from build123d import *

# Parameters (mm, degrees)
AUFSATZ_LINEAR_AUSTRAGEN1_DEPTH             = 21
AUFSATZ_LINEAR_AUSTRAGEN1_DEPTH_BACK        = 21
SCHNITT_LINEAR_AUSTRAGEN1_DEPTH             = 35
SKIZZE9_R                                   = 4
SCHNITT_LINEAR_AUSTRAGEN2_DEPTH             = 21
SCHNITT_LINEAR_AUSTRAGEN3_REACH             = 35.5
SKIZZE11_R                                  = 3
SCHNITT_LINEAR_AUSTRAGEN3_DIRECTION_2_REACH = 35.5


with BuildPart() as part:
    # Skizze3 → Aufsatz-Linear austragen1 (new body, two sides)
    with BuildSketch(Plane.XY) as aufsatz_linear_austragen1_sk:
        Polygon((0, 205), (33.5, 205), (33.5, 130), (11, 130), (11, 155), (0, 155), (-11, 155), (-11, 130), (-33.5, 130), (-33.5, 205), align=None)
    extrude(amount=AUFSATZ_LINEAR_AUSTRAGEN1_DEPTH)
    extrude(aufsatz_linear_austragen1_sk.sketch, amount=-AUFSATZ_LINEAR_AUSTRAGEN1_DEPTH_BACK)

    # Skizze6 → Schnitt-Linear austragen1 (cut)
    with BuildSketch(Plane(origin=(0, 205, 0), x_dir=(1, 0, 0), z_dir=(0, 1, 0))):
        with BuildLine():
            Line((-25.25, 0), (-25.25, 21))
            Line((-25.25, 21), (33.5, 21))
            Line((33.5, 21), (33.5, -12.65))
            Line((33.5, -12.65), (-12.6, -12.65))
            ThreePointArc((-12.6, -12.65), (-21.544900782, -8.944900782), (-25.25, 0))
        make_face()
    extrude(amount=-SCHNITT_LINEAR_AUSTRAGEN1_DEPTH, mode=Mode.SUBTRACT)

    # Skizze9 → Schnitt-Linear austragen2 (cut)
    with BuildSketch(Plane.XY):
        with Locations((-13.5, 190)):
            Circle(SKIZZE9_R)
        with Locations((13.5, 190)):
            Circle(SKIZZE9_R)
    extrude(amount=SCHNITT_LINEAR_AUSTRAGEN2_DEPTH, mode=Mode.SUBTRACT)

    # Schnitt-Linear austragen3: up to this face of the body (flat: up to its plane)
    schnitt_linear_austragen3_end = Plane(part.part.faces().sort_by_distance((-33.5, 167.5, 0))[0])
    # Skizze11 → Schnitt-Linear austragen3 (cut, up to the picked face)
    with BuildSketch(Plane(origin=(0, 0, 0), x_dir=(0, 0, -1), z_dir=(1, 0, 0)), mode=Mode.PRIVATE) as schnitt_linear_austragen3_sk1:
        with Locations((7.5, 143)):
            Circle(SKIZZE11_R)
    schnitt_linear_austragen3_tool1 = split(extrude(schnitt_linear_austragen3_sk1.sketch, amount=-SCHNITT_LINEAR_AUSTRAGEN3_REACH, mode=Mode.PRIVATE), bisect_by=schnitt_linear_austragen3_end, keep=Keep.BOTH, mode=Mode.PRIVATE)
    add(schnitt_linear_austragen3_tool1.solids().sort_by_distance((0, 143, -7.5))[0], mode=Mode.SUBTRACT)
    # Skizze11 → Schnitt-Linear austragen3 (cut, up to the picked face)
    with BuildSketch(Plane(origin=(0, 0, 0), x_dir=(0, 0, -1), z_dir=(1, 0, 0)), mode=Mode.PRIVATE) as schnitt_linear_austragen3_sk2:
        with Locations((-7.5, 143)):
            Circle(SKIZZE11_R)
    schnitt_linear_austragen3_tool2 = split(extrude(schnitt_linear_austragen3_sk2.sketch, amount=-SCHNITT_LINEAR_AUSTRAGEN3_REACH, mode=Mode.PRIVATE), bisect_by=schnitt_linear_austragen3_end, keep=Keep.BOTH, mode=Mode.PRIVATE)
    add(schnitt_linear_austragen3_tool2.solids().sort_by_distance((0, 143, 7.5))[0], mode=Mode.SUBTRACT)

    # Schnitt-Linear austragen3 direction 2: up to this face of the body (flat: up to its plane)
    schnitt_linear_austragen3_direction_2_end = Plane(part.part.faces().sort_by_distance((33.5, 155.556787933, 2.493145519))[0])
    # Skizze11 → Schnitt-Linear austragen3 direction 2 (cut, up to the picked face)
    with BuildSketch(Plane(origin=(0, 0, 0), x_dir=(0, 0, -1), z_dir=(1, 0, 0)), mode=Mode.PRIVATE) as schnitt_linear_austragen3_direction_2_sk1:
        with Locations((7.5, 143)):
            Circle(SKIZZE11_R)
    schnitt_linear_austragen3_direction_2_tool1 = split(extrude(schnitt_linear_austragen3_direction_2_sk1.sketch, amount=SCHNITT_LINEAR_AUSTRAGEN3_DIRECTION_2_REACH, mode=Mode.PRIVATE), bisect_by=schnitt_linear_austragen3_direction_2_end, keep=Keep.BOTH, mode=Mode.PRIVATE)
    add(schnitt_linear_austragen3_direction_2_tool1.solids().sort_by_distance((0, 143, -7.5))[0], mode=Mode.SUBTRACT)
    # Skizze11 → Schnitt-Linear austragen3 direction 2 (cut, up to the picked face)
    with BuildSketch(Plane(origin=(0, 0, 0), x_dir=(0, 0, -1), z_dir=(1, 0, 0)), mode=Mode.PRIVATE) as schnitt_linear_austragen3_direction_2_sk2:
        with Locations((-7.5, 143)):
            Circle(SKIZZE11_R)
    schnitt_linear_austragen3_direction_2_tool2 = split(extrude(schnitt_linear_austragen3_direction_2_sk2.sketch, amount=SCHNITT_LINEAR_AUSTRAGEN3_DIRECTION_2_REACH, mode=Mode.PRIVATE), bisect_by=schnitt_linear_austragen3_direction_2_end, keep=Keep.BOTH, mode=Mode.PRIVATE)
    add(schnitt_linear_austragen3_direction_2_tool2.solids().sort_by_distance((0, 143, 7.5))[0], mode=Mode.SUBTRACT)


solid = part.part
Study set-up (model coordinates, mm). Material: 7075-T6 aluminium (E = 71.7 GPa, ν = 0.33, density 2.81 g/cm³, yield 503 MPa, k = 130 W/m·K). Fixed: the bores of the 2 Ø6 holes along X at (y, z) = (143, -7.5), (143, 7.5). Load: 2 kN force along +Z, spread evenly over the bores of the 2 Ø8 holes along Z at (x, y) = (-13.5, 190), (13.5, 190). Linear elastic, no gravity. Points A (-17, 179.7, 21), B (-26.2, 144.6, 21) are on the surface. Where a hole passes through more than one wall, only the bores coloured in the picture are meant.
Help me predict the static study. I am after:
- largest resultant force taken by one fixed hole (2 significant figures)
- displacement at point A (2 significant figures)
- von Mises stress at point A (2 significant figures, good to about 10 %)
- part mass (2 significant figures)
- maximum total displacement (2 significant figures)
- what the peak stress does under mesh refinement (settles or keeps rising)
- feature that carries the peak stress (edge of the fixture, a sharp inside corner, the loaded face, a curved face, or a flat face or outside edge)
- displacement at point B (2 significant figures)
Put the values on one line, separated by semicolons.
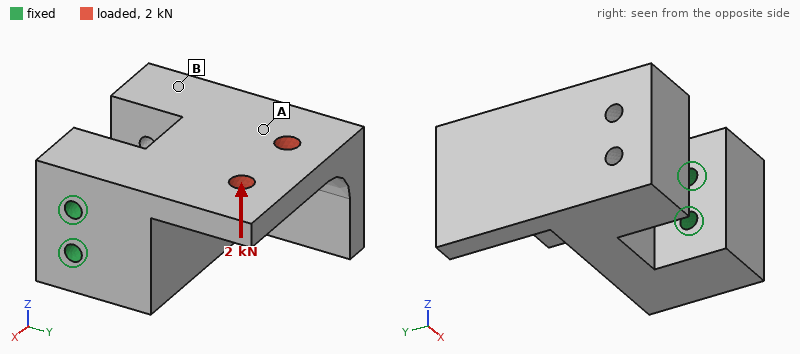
5.0 kN; 41 µm; 16 MPa; 330 g; 87 µm; keeps rising; edge of the fixture; 18 µm
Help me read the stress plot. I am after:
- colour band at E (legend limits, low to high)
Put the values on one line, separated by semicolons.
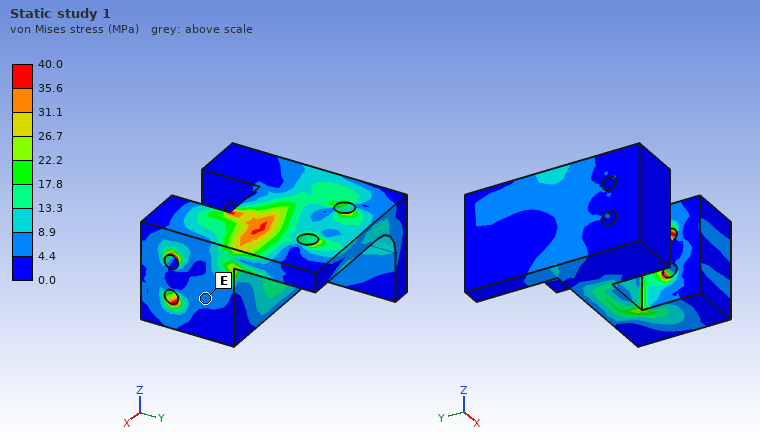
4.4 to 8.9 MPa
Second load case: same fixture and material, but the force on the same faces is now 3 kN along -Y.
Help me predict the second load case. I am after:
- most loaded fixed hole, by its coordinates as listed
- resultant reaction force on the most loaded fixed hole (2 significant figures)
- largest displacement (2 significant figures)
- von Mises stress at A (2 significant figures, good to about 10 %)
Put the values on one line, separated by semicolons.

(143, 7.5); 4.1 kN; 80 µm; 6.9 MPa
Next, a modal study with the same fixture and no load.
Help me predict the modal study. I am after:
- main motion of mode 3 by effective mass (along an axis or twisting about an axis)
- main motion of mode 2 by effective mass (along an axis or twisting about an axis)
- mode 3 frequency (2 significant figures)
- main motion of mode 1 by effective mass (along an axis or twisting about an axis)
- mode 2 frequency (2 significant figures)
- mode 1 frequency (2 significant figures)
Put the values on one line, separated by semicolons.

twisting about X; along Z; 3200 Hz; along Y; 2800 Hz; 2000 Hz
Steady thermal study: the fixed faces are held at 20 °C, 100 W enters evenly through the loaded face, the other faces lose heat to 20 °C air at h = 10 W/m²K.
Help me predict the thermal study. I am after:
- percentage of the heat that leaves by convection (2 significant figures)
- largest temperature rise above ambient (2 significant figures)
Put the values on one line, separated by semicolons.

6.7 %; 63 K
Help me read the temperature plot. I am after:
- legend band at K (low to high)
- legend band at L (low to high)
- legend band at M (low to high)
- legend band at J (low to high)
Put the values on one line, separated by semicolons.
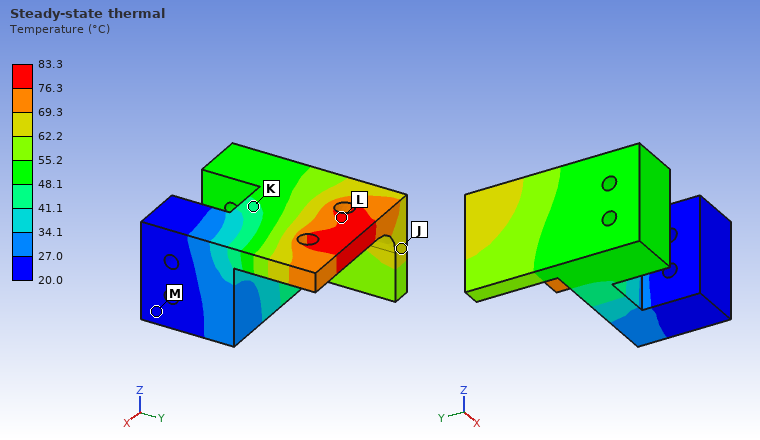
41.1 to 48.1 °C; 76.3 to 83.3 °C; 20.0 to 27.0 °C; 62.2 to 69.3 °C
